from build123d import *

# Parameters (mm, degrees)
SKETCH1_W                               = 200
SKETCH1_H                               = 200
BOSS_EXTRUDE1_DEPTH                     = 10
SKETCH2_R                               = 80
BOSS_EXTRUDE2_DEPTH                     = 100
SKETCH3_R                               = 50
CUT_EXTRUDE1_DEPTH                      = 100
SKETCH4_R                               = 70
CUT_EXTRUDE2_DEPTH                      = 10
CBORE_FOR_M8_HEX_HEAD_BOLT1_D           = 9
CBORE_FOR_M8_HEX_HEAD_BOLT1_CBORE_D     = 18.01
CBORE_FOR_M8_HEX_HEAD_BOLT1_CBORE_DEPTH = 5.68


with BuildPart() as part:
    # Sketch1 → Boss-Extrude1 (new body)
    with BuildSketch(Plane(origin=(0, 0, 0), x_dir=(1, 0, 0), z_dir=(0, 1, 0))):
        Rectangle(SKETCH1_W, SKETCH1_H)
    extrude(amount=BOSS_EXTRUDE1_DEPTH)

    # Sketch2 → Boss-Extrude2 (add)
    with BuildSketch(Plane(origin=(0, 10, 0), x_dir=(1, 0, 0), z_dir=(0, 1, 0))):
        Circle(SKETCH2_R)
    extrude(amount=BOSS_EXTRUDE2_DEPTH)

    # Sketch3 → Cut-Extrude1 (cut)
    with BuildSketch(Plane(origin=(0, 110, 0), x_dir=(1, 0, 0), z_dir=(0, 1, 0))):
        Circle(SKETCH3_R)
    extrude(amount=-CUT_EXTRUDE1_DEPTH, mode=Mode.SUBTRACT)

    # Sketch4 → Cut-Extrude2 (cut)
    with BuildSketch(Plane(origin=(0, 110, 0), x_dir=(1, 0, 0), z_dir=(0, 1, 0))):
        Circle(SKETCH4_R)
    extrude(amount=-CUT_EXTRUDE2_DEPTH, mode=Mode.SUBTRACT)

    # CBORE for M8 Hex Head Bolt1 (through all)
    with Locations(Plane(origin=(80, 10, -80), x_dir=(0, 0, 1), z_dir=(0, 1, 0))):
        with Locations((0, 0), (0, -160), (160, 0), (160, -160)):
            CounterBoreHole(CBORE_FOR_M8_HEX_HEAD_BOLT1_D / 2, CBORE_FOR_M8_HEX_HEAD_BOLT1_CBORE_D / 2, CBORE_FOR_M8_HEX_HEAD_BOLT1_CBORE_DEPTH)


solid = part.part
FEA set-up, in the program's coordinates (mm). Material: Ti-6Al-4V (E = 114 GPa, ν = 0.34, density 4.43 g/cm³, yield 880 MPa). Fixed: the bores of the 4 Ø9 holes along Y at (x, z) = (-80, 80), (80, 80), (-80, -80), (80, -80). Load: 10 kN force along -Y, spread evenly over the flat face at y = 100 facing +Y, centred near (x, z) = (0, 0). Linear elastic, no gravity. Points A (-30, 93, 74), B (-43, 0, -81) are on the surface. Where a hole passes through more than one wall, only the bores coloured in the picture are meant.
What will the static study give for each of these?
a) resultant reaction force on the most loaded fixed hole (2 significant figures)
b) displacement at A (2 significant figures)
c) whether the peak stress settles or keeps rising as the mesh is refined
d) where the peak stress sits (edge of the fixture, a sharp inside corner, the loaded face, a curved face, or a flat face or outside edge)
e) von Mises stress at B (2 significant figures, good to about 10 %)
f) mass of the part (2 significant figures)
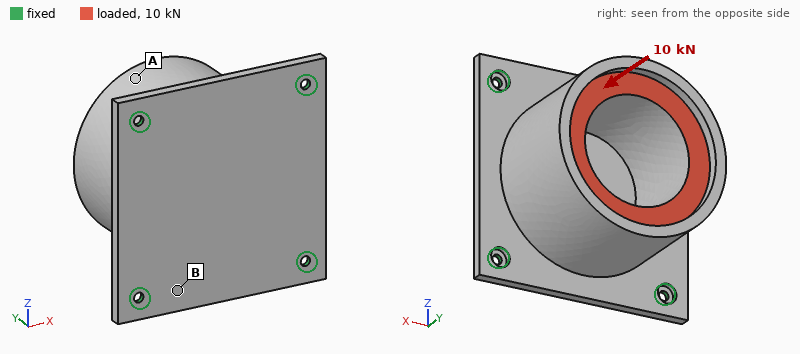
4.2 kN
42 µm
keeps rising
edge of the fixture
17 MPa
6.8 kg
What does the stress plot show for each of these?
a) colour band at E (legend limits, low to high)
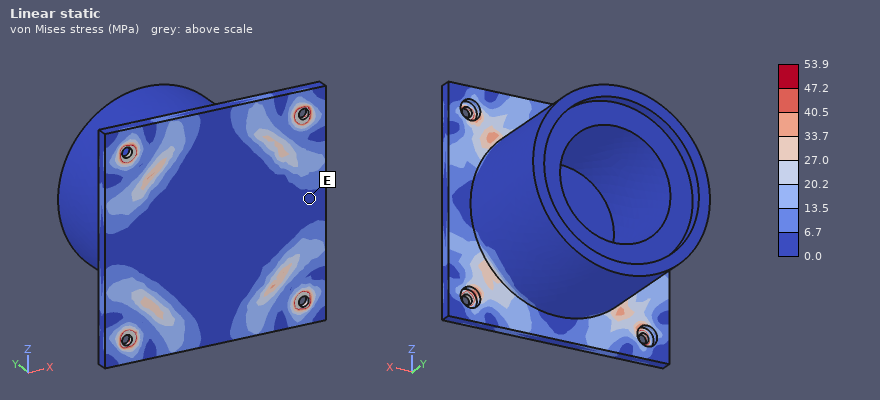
0.0 to 6.7 MPa
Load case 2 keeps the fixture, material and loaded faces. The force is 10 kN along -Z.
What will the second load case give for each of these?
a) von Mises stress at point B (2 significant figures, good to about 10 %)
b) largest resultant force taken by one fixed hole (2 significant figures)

26 MPa
5.1 kN
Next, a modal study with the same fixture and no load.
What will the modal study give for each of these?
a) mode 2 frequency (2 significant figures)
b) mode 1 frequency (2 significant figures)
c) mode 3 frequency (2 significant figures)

990 Hz
960 Hz
990 Hz
